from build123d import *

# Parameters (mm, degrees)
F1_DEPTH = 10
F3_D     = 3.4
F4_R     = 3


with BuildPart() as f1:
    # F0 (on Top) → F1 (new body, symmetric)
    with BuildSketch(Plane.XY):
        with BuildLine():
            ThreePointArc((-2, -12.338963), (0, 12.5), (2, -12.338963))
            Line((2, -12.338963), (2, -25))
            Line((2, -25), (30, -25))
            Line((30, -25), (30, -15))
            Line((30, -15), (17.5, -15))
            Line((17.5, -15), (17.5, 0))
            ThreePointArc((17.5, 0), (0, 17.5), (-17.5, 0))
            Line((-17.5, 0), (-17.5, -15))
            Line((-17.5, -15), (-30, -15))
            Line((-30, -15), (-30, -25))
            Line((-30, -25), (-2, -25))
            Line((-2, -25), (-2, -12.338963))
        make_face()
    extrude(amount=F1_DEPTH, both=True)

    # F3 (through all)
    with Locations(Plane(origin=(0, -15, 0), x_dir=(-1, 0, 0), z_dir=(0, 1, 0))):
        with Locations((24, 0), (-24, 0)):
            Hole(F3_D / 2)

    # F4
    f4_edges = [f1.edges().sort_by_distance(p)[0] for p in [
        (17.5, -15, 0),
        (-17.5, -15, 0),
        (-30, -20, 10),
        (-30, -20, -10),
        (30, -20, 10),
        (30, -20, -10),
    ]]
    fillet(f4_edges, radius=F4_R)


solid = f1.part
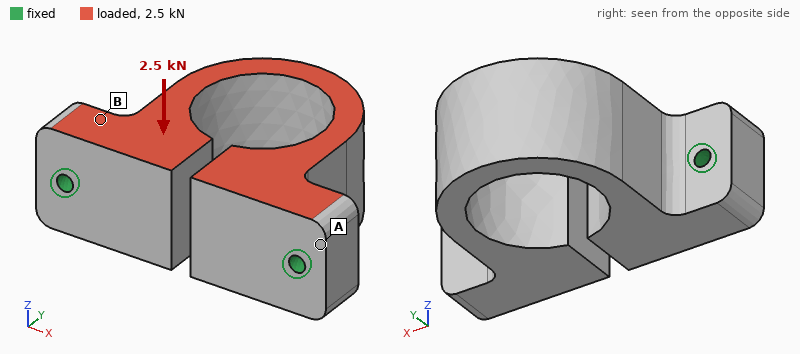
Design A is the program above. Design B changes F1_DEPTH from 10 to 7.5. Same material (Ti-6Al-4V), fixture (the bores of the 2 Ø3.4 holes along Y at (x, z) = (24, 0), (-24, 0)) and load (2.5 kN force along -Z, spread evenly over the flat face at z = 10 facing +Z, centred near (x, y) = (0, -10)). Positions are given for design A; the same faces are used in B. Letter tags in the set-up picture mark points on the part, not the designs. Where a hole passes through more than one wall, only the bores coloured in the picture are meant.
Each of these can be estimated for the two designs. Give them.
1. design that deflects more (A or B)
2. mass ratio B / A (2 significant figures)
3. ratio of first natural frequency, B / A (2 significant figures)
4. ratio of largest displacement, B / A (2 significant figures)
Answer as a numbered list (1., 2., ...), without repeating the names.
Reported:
1. B
2. 0.75
3. 0.98
4. 1.4
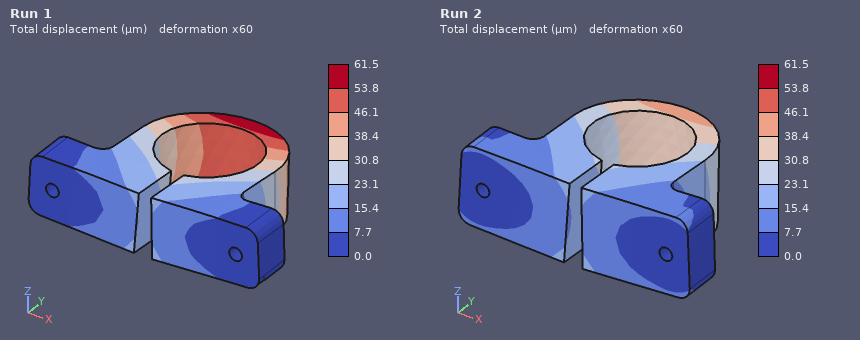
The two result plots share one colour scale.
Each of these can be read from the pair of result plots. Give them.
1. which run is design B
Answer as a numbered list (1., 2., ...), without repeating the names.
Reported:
1. Run 1
